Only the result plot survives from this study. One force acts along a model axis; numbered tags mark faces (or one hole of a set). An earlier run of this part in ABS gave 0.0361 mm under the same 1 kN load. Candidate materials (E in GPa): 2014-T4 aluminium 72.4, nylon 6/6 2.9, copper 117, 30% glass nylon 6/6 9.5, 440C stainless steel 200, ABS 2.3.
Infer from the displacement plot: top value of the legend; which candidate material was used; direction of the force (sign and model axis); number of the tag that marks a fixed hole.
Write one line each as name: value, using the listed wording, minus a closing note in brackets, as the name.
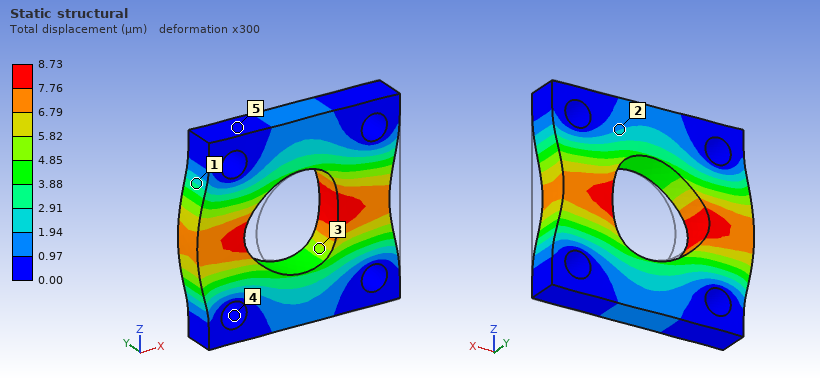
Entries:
top value of the legend: 8.73 µm
which candidate material was used: 30% glass nylon 6/6
direction of the force: -X
number of the tag that marks a fixed hole: 4
